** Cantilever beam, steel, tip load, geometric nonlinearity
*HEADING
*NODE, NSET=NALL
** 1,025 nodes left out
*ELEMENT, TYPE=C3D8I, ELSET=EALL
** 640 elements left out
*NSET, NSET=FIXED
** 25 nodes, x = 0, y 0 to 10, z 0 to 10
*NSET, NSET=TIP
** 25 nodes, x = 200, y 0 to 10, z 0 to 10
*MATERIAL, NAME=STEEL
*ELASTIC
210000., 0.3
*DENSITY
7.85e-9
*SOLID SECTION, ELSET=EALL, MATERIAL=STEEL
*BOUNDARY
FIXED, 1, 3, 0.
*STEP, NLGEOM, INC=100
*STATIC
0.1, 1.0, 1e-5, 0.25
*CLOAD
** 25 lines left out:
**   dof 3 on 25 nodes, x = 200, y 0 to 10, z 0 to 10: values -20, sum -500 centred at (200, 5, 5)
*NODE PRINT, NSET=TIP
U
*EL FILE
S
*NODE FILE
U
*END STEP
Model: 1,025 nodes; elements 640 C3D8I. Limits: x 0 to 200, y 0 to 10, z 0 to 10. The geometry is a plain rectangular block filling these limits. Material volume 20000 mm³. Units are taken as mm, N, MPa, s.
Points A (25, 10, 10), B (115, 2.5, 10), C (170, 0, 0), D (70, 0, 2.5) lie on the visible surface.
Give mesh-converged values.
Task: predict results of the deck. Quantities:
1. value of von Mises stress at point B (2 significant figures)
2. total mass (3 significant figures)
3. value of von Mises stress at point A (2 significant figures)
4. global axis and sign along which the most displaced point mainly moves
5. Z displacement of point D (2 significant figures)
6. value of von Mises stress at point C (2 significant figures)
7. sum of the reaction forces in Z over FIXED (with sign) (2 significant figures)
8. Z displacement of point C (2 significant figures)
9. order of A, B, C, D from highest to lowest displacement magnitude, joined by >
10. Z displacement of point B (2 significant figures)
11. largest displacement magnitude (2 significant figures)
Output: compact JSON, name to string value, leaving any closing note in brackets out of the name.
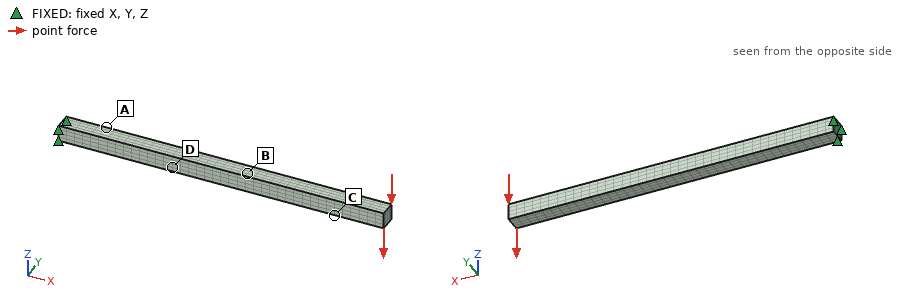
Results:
{"value of von Mises stress at point B": "260 MPa", "total mass": "0.157 kg", "value of von Mises stress at point A": "530 MPa", "global axis and sign along which the most displaced point mainly moves": "-Z", "Z displacement of point D": "-1.2 mm", "value of von Mises stress at point C": "90 MPa", "sum of the reaction forces in Z over FIXED (with sign)": "500 N", "Z displacement of point C": "-5.9 mm", "order of A, B, C, D from highest to lowest displacement magnitude, joined by >": "C > B > D > A", "Z displacement of point B": "-3.0 mm", "largest displacement magnitude": "7.6 mm"}
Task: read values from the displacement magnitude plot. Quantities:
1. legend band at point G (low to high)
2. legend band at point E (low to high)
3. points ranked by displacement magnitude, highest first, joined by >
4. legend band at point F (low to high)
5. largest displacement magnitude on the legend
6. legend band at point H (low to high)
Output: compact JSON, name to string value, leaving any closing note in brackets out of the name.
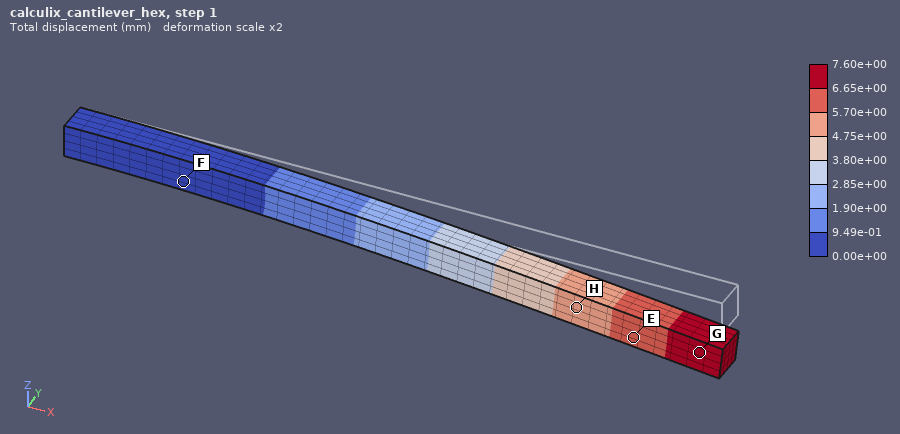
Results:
{"legend band at point G": "6.65e+00 to 7.60e+00 mm", "legend band at point E": "5.70e+00 to 6.65e+00 mm", "points ranked by displacement magnitude, highest first, joined by >": "G > E > H > F", "legend band at point F": "0.00e+00 to 9.49e-01 mm", "largest displacement magnitude on the legend": "7.60e+00 mm", "legend band at point H": "4.75e+00 to 5.70e+00 mm"}
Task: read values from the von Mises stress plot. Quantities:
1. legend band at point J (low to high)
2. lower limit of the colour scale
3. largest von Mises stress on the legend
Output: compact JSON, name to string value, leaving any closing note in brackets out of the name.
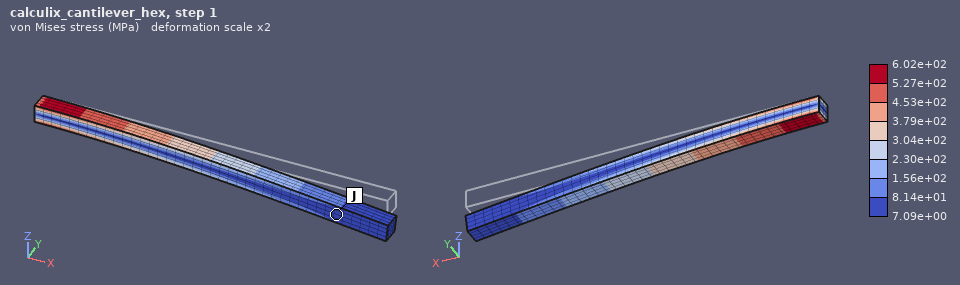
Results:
{"legend band at point J": "7.09e+00 to 8.14e+01 MPa", "lower limit of the colour scale": "7.09e+00 MPa", "largest von Mises stress on the legend": "6.02e+02 MPa"}
